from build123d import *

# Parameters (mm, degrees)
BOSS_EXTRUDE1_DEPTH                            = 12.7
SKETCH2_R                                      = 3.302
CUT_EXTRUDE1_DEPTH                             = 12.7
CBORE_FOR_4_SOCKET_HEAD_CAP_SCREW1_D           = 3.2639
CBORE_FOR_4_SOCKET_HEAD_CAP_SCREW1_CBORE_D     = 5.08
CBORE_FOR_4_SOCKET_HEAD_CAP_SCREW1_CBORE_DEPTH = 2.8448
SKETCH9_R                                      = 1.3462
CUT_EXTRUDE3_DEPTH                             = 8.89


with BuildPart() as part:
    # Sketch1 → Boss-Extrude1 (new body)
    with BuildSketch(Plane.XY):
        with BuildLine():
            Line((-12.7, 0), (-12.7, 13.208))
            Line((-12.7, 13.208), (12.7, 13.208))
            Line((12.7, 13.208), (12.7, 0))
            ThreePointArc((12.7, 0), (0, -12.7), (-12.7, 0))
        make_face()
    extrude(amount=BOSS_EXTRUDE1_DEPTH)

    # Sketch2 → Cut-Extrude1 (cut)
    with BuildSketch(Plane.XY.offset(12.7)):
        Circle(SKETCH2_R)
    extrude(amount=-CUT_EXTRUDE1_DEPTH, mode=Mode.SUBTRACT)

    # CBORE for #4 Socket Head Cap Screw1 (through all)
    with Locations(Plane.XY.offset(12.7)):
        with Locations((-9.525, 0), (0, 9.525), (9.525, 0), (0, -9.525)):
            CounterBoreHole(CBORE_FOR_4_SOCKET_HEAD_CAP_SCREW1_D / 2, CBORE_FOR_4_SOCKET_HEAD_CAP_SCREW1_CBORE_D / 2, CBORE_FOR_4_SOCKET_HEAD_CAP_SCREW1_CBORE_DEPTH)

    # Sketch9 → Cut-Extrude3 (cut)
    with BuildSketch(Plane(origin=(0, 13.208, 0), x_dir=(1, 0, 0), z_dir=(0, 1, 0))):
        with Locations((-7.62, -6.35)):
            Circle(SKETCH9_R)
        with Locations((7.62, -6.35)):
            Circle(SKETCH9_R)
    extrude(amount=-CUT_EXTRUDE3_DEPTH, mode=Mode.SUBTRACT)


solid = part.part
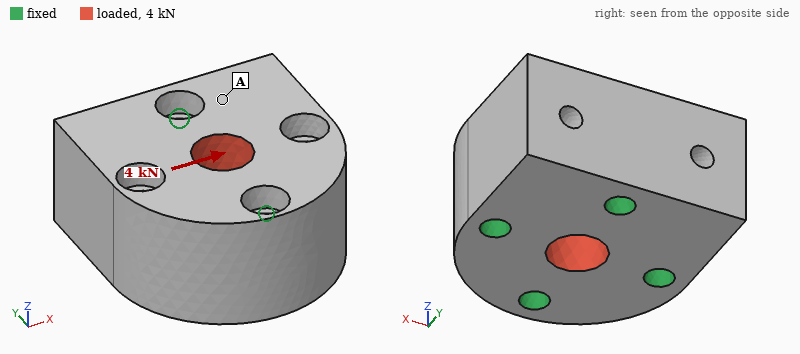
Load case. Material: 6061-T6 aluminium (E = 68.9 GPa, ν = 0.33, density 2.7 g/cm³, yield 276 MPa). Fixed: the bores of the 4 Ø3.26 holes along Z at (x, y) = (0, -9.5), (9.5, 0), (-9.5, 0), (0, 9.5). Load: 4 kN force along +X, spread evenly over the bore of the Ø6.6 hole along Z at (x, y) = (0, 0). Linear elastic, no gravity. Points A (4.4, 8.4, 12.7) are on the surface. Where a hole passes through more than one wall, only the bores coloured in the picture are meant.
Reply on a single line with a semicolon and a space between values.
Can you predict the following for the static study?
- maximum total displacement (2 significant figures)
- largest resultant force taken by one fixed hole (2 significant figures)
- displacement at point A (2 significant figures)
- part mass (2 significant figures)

2.5 µm; 1.3 kN; 0.85 µm; 17 g
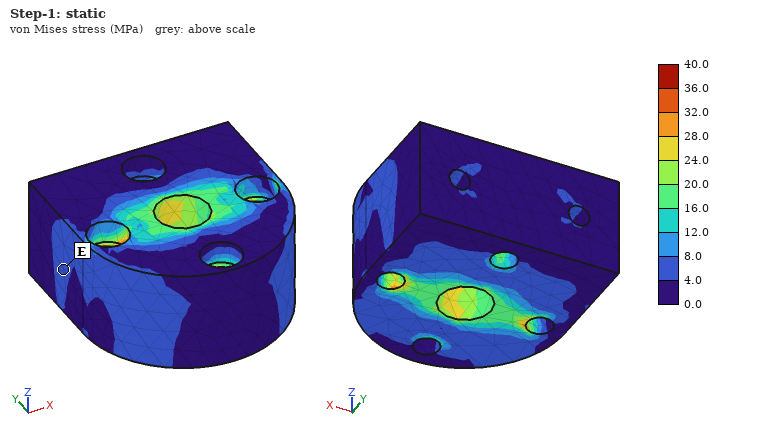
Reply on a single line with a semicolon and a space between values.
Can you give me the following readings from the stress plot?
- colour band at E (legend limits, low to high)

4.0 to 8.0 MPa
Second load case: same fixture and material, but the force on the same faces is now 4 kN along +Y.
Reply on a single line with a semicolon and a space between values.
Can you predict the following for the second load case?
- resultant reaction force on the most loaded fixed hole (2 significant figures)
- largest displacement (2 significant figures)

1.3 kN; 2.5 µm
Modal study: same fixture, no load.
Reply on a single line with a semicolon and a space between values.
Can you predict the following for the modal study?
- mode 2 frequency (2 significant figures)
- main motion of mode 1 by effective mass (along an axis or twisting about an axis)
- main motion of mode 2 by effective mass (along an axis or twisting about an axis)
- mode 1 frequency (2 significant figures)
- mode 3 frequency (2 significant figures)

56 kHz; twisting about Y; along Z; 53 kHz; 80 kHz
